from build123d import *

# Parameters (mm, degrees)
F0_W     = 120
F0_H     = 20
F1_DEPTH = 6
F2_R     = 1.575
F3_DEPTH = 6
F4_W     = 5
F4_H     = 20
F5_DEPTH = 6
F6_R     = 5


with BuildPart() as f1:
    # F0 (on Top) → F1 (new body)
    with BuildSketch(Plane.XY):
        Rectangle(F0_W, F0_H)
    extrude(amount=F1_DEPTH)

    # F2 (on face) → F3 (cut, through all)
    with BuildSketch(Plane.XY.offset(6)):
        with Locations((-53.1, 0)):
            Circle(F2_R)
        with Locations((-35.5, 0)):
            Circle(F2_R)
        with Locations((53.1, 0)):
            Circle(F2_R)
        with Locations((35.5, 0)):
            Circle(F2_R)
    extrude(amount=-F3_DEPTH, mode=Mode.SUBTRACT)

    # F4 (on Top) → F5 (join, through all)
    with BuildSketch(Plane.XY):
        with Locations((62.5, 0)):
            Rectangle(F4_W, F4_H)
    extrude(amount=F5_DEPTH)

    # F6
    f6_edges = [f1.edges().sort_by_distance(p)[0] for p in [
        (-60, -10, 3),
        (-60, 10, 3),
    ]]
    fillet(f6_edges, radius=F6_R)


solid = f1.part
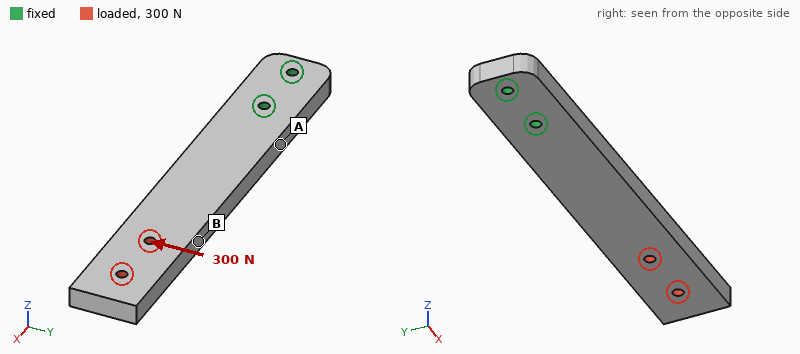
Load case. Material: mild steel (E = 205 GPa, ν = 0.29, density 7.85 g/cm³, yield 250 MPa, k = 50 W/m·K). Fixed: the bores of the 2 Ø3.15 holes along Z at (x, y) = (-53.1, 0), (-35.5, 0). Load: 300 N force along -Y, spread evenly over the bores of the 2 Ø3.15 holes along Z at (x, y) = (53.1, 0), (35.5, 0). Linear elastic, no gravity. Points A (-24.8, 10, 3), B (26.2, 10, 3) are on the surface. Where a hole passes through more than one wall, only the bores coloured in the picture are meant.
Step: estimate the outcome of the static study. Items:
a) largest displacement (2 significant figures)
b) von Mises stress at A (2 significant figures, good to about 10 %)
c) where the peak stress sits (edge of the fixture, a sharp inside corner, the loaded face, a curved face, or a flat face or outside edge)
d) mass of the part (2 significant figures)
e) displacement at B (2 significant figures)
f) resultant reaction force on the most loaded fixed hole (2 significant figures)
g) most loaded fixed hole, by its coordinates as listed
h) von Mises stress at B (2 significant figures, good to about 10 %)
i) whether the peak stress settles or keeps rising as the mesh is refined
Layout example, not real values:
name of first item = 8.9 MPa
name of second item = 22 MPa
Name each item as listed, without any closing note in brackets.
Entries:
largest displacement = 0.12 mm
von Mises stress at A = 53 MPa
where the peak stress sits = edge of the fixture
mass of the part = 120 g
displacement at B = 0.063 mm
resultant reaction force on the most loaded fixed hole = 1.4 kN
most loaded fixed hole, by its coordinates as listed = (-35.5, 0)
von Mises stress at B = 14 MPa
whether the peak stress settles or keeps rising as the mesh is refined = keeps rising
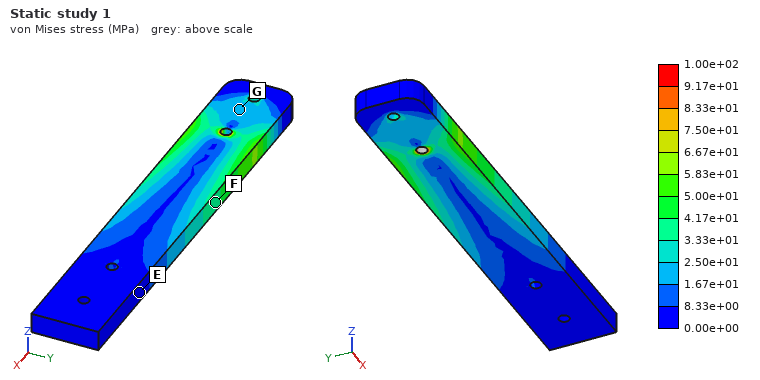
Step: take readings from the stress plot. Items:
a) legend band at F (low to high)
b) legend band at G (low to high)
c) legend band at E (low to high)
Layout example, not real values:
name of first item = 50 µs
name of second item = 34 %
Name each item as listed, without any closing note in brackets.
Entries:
legend band at F = 3.33e+01 to 4.17e+01 MPa
legend band at G = 1.67e+01 to 2.50e+01 MPa
legend band at E = 0.00e+00 to 8.33e+00 MPa
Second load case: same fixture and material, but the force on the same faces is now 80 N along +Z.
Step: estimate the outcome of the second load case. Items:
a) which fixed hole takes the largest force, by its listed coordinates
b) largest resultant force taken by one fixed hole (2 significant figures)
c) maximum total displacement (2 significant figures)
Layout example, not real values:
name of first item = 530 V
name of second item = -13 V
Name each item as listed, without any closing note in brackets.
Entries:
which fixed hole takes the largest force, by its listed coordinates = (-35.5, 0)
largest resultant force taken by one fixed hole = 220 N
maximum total displacement = 0.26 mm
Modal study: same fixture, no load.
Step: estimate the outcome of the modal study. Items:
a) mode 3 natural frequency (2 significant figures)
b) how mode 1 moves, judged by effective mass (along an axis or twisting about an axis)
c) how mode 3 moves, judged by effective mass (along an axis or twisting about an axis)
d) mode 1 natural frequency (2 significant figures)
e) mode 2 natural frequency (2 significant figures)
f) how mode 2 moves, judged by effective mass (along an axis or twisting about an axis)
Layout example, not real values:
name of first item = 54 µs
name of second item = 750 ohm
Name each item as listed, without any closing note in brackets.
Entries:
mode 3 natural frequency = 3000 Hz
how mode 1 moves, judged by effective mass = along Z
how mode 3 moves, judged by effective mass = along Z
mode 1 natural frequency = 480 Hz
mode 2 natural frequency = 1400 Hz
how mode 2 moves, judged by effective mass = along Y
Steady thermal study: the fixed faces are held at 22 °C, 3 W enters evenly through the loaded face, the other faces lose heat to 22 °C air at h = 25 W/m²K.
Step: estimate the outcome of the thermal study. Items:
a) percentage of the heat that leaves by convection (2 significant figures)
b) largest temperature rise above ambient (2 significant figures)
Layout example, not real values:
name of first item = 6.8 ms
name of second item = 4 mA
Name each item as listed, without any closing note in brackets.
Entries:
percentage of the heat that leaves by convection = 56 %
largest temperature rise above ambient = 23 K
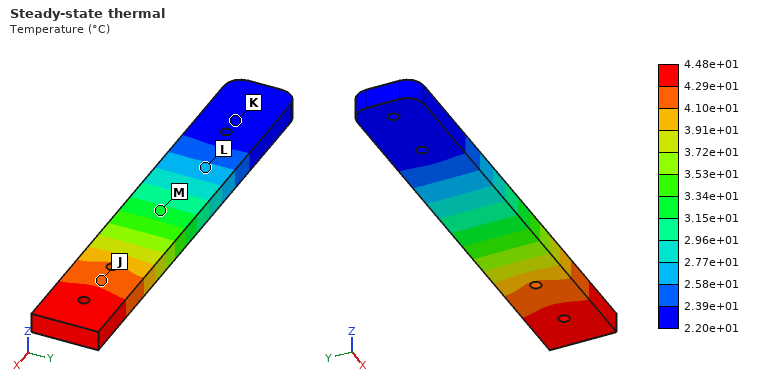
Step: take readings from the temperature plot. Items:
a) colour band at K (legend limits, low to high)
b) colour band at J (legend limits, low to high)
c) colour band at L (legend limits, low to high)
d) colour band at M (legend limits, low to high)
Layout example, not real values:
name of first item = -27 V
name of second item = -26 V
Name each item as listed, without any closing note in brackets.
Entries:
colour band at K = 2.20e+01 to 2.39e+01 °C
colour band at J = 4.10e+01 to 4.29e+01 °C
colour band at L = 2.58e+01 to 2.77e+01 °C
colour band at M = 3.15e+01 to 3.34e+01 °C
